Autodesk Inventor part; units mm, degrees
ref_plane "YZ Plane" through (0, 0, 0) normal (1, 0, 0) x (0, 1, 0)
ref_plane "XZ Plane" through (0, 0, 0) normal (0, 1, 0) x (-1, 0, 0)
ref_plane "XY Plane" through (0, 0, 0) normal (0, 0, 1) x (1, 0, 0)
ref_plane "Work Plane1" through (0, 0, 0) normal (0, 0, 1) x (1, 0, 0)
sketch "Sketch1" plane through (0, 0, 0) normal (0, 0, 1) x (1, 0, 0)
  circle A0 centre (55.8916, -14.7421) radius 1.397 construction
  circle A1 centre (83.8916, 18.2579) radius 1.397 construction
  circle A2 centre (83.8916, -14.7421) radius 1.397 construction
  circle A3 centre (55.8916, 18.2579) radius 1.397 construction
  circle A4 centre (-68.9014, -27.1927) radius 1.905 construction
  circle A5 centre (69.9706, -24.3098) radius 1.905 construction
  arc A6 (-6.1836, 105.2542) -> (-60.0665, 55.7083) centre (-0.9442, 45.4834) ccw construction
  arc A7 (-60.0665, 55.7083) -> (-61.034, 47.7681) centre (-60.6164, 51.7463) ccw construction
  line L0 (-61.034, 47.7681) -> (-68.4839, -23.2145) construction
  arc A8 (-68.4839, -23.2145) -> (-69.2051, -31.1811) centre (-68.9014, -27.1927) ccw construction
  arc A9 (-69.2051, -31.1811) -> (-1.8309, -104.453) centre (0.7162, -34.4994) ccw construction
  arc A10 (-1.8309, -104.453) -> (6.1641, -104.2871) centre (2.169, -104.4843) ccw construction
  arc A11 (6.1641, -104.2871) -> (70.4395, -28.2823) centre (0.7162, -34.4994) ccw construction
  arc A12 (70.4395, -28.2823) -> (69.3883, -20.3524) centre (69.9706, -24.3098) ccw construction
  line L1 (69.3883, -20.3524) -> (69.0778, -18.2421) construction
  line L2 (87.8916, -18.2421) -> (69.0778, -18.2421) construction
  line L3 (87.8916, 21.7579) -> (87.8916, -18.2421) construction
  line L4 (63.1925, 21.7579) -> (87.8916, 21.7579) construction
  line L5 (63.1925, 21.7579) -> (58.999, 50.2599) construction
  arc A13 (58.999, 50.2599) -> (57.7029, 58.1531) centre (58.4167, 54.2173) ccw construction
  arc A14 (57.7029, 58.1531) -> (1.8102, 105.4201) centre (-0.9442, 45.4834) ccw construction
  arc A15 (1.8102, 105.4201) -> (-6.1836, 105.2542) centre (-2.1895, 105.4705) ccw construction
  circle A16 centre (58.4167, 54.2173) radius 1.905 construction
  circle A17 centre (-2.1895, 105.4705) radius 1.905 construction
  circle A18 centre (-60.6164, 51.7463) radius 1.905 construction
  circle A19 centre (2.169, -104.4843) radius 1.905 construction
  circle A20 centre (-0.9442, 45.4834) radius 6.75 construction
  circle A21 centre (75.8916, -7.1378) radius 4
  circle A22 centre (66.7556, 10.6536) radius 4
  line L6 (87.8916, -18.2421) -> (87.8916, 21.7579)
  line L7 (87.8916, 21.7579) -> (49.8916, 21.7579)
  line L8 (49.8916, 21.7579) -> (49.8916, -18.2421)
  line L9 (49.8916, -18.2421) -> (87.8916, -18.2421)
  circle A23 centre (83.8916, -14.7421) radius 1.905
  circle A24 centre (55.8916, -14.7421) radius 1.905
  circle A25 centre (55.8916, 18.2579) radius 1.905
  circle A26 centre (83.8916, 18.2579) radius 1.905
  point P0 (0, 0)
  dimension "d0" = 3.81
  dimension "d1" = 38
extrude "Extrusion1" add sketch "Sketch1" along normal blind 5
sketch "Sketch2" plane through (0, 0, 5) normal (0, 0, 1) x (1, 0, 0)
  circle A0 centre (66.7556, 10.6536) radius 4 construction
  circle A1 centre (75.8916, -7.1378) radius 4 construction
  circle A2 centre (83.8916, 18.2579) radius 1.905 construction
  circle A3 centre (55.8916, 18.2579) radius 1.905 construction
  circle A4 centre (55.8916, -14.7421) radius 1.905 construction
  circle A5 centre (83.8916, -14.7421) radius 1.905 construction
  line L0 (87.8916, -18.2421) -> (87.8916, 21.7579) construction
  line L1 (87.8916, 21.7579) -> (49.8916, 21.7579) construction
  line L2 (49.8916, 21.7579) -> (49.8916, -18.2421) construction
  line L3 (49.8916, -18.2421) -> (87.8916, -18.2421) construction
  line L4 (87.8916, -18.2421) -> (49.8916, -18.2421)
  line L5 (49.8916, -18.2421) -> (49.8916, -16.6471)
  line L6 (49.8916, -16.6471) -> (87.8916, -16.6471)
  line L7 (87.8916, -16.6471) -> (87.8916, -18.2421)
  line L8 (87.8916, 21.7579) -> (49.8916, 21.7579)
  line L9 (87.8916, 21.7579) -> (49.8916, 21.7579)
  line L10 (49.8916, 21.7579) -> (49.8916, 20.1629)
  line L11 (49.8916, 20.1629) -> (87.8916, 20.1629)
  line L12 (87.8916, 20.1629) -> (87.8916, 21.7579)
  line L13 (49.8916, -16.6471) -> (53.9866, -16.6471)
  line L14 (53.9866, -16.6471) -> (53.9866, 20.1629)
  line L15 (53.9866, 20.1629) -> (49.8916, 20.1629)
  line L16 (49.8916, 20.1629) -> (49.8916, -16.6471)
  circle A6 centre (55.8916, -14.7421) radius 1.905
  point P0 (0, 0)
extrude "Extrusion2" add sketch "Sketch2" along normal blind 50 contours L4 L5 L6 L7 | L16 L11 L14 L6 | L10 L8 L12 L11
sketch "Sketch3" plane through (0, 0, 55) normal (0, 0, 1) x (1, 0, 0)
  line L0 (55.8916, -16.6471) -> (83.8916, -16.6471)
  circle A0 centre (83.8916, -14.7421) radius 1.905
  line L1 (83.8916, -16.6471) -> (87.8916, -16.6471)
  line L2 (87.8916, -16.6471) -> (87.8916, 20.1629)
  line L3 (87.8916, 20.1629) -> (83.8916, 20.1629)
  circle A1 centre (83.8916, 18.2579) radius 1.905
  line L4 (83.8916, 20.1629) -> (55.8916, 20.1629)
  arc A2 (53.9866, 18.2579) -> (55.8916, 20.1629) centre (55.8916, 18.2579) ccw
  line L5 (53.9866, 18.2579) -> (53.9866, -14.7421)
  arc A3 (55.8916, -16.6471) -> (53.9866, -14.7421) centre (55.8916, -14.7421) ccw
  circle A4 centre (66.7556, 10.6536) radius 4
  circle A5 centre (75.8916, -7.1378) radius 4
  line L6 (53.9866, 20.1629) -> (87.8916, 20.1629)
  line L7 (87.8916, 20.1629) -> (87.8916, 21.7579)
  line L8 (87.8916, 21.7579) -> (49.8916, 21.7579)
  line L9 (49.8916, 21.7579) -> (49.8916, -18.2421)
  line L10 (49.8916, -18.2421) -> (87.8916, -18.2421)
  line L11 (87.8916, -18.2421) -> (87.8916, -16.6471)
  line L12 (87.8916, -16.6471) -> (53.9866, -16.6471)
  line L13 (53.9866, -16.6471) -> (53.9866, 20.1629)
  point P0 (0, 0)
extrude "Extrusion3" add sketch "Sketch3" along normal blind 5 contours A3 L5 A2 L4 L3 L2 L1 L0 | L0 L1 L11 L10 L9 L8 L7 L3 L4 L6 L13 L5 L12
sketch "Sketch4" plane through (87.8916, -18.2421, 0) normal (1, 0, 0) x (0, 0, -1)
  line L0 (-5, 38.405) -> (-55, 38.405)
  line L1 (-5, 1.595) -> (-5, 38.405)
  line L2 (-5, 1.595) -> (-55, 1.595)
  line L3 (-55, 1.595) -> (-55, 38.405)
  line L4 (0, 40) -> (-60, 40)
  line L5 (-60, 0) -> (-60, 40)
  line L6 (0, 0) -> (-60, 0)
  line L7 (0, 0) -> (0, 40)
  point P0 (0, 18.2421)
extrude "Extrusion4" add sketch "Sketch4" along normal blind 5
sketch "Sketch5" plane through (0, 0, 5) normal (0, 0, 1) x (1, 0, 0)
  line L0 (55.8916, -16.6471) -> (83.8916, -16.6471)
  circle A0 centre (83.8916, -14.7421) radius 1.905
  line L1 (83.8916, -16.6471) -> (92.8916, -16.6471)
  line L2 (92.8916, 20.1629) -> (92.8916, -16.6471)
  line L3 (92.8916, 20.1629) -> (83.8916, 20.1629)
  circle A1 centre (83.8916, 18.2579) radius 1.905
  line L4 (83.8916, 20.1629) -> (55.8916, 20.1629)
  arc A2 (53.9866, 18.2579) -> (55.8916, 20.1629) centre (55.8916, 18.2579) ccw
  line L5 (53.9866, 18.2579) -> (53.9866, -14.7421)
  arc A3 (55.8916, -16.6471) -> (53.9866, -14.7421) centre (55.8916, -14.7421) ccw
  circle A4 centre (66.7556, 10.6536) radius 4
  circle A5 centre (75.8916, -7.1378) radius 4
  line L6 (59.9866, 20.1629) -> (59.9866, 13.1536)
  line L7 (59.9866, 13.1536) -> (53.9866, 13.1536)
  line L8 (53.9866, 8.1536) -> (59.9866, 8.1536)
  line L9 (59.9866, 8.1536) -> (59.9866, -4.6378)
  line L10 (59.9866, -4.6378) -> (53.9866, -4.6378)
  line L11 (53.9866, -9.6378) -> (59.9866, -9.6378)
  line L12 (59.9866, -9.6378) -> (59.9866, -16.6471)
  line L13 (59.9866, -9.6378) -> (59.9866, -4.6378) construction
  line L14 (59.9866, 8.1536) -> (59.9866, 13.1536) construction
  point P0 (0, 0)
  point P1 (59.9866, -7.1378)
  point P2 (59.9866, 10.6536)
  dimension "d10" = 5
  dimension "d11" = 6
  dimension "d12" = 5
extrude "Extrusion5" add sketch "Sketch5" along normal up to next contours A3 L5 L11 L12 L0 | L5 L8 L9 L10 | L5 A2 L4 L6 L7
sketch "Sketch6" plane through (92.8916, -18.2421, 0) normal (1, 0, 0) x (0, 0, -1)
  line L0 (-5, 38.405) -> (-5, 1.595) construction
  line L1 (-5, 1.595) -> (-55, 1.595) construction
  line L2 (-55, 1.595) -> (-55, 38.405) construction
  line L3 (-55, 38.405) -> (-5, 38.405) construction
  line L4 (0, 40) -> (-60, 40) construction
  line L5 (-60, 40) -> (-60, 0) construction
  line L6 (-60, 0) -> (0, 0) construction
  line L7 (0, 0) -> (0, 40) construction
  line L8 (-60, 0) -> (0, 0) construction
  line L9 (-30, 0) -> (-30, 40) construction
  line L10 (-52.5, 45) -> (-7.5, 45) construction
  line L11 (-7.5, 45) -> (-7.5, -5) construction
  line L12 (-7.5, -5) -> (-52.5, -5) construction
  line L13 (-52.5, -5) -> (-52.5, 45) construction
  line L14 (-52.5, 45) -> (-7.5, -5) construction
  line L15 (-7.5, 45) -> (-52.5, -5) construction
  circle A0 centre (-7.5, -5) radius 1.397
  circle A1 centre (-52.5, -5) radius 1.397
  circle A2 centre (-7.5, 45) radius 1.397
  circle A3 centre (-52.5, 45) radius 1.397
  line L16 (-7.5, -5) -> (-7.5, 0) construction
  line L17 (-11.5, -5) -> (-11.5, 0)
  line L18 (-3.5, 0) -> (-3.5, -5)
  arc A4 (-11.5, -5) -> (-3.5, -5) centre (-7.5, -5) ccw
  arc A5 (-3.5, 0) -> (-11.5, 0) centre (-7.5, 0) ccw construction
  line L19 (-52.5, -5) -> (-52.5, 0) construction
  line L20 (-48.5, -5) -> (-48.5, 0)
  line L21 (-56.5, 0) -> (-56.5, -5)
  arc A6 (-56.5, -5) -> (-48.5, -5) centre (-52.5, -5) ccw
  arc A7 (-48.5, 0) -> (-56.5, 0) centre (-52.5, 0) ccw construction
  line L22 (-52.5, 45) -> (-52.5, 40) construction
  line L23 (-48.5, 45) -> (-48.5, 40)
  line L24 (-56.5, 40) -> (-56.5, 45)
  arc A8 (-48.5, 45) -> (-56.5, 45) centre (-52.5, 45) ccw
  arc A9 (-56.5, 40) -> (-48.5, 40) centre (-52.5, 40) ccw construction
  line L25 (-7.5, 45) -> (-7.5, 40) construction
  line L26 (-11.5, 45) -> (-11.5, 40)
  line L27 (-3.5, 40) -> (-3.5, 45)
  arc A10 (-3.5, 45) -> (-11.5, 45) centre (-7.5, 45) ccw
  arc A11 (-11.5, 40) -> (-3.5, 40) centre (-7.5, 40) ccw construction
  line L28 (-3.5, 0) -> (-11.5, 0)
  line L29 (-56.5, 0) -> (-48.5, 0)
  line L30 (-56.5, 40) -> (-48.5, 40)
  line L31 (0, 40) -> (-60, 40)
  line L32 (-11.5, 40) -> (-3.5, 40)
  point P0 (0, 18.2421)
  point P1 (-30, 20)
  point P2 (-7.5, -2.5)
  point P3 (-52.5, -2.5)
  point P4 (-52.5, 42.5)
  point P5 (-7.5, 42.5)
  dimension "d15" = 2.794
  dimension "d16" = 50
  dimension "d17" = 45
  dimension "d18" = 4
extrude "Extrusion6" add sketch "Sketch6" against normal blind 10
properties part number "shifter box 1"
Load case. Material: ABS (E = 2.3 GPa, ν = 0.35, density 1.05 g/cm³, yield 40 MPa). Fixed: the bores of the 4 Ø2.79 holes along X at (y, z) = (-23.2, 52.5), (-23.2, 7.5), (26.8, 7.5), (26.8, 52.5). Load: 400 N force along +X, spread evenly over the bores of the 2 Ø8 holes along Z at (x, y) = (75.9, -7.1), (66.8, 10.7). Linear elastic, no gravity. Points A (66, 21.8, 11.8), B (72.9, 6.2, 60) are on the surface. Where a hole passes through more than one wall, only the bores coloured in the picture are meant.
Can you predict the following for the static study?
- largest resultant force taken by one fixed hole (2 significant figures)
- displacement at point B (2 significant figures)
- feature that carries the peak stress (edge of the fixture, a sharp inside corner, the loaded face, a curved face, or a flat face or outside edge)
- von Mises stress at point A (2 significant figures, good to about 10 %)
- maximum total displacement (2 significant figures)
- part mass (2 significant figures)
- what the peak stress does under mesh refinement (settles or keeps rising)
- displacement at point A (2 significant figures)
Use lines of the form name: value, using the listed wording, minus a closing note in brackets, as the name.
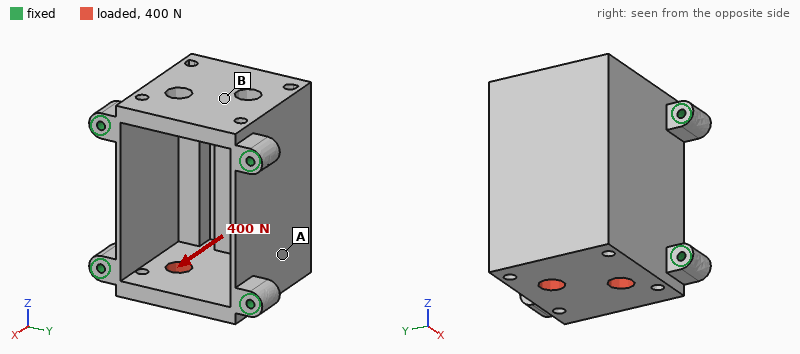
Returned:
largest resultant force taken by one fixed hole: 220 N
displacement at point B: 0.025 mm
feature that carries the peak stress: edge of the fixture
von Mises stress at point A: 1.5 MPa
maximum total displacement: 0.10 mm
part mass: 41 g
what the peak stress does under mesh refinement: keeps rising
displacement at point A: 0.058 mm
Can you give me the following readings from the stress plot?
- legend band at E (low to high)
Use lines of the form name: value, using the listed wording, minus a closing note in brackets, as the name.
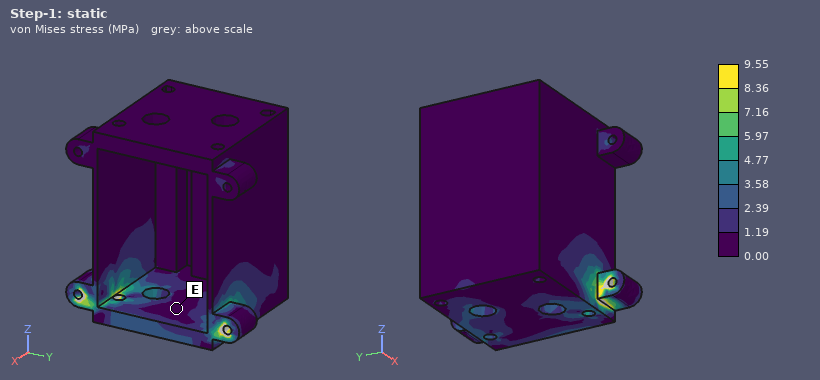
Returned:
legend band at E: 0.00 to 1.19 MPa
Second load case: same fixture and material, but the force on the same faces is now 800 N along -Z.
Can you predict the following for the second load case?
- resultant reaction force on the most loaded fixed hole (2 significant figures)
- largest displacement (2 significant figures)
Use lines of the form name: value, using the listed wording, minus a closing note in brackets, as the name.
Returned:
resultant reaction force on the most loaded fixed hole: 360 N
largest displacement: 0.49 mm
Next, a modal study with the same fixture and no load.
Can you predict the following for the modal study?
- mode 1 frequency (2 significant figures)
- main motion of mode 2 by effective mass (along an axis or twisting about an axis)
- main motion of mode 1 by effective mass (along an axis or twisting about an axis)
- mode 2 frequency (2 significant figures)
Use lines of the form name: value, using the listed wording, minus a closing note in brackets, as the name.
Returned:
mode 1 frequency: 1500 Hz
main motion of mode 2 by effective mass: along Y
main motion of mode 1 by effective mass: along Z
mode 2 frequency: 1600 Hz
